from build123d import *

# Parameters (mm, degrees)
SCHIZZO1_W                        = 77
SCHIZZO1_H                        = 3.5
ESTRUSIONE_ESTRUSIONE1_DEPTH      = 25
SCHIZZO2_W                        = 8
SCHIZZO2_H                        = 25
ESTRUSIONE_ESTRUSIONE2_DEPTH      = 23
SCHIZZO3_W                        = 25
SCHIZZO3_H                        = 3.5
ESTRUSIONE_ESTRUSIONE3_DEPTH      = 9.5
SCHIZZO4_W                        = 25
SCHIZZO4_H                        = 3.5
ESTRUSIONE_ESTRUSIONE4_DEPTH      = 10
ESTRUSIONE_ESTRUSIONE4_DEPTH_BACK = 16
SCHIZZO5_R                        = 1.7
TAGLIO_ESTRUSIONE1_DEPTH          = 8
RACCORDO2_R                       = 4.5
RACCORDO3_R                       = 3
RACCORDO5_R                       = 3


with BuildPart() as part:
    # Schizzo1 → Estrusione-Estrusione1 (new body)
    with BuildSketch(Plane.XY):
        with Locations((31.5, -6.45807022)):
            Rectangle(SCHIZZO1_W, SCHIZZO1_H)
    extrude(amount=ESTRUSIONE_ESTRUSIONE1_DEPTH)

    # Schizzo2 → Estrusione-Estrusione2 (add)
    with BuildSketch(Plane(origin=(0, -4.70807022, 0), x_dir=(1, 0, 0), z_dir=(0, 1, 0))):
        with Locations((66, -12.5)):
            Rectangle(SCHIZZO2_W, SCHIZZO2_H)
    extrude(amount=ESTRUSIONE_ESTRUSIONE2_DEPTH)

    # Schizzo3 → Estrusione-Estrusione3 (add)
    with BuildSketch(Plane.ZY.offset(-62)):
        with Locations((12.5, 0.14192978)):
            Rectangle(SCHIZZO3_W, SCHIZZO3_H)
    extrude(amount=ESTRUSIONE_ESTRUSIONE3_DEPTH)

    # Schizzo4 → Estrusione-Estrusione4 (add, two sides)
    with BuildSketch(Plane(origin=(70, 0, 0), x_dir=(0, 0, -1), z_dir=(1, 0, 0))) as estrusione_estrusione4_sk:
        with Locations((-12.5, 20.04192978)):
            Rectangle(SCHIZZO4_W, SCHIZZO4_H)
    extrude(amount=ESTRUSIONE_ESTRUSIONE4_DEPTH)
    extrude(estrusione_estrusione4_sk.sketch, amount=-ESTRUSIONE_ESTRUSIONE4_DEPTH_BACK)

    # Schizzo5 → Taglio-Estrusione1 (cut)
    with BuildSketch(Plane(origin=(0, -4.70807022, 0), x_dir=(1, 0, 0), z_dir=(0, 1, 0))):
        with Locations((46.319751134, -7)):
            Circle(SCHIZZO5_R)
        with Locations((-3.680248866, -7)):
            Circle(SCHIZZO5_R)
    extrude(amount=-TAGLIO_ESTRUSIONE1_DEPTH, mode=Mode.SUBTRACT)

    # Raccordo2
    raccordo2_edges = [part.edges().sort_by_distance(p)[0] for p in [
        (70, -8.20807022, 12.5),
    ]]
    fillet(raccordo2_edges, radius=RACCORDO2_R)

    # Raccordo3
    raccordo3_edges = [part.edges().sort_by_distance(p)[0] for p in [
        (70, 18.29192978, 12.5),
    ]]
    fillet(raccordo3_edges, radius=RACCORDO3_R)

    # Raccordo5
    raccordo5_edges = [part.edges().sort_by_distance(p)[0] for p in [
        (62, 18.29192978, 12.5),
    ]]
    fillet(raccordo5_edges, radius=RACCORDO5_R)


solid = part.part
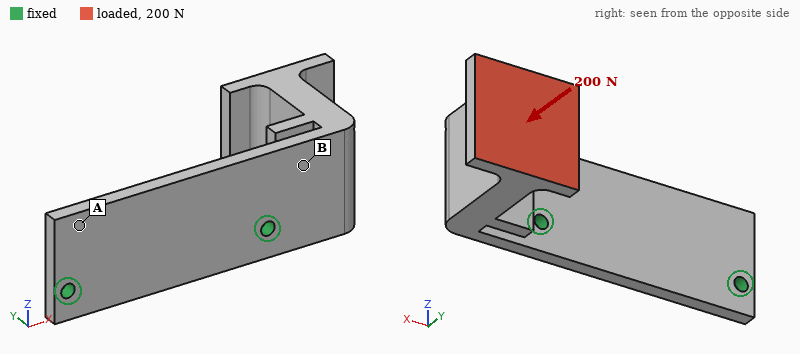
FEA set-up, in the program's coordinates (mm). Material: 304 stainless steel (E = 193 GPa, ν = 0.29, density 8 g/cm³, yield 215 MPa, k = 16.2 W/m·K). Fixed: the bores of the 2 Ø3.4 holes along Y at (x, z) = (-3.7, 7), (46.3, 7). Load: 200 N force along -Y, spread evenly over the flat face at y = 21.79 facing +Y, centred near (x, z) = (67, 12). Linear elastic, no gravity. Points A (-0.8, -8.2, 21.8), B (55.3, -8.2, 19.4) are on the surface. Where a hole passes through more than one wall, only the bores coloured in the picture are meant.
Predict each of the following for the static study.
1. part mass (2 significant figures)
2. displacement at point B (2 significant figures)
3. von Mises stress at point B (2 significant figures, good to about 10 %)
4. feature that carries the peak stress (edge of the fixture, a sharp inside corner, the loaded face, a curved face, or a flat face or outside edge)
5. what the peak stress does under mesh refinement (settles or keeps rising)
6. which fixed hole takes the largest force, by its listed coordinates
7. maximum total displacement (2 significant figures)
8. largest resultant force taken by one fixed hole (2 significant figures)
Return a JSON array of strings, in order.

["110 g", "0.018 mm", "37 MPa", "edge of the fixture", "keeps rising", "(46.3, 7)", "0.12 mm", "220 N"]
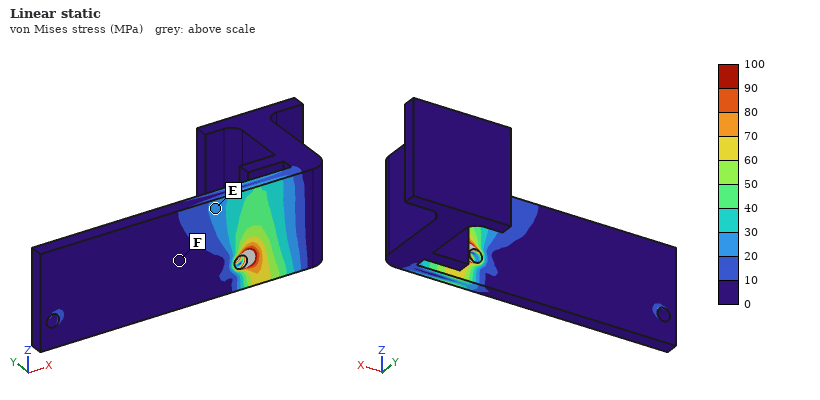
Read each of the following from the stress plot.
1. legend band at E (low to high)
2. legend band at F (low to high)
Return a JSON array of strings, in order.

["20 to 30 MPa", "0 to 10 MPa"]
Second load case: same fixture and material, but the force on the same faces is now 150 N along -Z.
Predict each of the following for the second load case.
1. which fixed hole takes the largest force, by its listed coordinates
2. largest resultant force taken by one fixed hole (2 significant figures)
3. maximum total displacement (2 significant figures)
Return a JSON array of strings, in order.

["(46.3, 7)", "220 N", "90 µm"]
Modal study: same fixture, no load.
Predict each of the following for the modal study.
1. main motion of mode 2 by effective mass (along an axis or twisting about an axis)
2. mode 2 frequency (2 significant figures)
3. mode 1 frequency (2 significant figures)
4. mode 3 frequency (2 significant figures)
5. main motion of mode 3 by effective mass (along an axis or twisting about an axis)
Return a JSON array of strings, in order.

["along Z", "1300 Hz", "840 Hz", "3500 Hz", "along Y"]
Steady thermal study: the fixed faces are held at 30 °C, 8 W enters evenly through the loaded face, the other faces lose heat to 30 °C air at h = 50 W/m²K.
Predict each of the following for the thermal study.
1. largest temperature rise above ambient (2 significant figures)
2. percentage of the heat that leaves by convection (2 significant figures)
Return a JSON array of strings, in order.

["63 K", "84 %"]
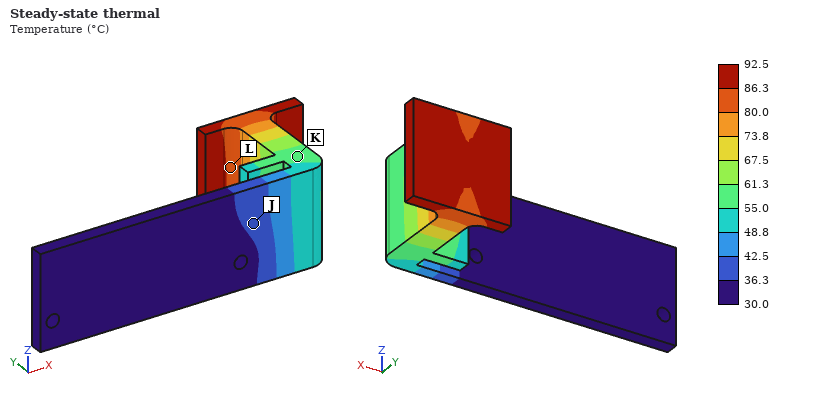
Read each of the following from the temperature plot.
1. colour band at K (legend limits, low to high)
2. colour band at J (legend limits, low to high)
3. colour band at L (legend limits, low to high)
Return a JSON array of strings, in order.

["55.0 to 61.3 °C", "36.3 to 42.5 °C", "80.0 to 86.3 °C"]
